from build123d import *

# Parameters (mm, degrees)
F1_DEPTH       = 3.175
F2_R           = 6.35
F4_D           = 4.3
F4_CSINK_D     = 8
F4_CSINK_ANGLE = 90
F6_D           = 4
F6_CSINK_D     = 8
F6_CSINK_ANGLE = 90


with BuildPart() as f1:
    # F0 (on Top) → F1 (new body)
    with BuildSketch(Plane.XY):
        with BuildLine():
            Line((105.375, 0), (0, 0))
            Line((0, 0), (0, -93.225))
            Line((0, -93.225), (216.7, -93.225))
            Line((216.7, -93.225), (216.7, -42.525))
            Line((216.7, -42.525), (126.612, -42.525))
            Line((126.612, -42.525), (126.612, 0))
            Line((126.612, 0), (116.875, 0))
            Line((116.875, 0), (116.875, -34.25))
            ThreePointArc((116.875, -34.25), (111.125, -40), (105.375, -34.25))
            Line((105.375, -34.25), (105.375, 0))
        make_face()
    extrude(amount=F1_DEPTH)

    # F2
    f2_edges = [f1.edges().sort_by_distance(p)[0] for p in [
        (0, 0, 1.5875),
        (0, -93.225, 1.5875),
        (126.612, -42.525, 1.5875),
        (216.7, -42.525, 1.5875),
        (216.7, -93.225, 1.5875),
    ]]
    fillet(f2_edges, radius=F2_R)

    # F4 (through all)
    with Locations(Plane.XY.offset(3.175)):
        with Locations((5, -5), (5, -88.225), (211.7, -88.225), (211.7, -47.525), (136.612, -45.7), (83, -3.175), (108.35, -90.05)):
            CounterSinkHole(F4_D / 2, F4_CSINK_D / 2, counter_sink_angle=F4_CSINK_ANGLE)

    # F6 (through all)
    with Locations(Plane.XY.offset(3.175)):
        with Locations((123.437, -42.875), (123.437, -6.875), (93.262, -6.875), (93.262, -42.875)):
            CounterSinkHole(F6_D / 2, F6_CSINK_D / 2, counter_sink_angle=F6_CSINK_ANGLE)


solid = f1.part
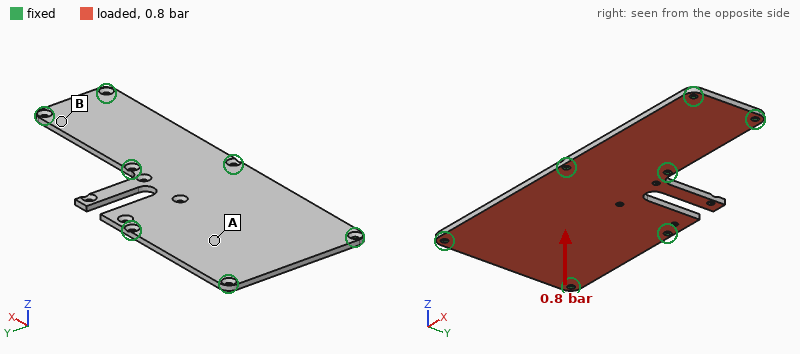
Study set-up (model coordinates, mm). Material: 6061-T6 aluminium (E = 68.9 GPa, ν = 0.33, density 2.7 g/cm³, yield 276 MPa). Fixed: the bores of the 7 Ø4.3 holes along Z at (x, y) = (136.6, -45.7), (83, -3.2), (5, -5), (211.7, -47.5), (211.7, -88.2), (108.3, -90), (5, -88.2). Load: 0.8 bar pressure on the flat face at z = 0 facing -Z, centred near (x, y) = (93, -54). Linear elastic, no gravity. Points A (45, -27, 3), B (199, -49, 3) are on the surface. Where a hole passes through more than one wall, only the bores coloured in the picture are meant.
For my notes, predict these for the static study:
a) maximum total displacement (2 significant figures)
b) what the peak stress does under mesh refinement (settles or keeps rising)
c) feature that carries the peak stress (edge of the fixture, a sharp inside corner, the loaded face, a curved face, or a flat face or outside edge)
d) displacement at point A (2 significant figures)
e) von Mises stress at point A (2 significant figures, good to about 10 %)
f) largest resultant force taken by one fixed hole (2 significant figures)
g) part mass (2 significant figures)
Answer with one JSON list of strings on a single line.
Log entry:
["0.30 mm", "keeps rising", "edge of the fixture", "0.18 mm", "21 MPa", "470 N", "130 g"]
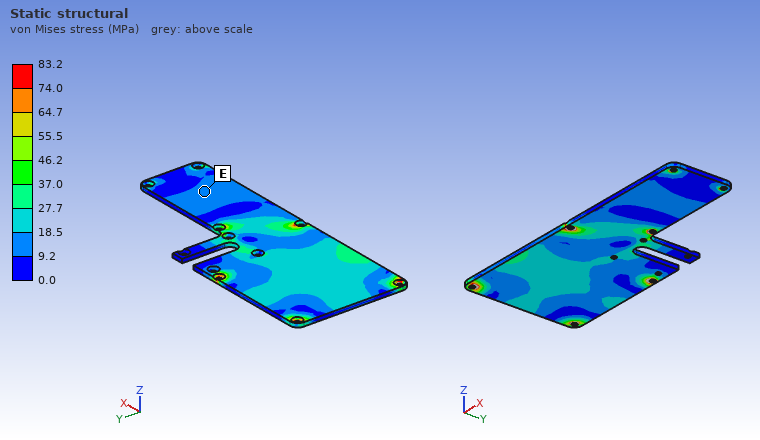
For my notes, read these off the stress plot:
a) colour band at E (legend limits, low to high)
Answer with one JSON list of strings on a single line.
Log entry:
["9.2 to 18.5 MPa"]
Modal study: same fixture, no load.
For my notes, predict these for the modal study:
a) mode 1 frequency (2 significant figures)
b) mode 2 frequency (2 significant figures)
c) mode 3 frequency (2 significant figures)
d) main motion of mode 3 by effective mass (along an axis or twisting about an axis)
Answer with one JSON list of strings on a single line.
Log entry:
["1100 Hz", "1200 Hz", "1700 Hz", "along Z"]
